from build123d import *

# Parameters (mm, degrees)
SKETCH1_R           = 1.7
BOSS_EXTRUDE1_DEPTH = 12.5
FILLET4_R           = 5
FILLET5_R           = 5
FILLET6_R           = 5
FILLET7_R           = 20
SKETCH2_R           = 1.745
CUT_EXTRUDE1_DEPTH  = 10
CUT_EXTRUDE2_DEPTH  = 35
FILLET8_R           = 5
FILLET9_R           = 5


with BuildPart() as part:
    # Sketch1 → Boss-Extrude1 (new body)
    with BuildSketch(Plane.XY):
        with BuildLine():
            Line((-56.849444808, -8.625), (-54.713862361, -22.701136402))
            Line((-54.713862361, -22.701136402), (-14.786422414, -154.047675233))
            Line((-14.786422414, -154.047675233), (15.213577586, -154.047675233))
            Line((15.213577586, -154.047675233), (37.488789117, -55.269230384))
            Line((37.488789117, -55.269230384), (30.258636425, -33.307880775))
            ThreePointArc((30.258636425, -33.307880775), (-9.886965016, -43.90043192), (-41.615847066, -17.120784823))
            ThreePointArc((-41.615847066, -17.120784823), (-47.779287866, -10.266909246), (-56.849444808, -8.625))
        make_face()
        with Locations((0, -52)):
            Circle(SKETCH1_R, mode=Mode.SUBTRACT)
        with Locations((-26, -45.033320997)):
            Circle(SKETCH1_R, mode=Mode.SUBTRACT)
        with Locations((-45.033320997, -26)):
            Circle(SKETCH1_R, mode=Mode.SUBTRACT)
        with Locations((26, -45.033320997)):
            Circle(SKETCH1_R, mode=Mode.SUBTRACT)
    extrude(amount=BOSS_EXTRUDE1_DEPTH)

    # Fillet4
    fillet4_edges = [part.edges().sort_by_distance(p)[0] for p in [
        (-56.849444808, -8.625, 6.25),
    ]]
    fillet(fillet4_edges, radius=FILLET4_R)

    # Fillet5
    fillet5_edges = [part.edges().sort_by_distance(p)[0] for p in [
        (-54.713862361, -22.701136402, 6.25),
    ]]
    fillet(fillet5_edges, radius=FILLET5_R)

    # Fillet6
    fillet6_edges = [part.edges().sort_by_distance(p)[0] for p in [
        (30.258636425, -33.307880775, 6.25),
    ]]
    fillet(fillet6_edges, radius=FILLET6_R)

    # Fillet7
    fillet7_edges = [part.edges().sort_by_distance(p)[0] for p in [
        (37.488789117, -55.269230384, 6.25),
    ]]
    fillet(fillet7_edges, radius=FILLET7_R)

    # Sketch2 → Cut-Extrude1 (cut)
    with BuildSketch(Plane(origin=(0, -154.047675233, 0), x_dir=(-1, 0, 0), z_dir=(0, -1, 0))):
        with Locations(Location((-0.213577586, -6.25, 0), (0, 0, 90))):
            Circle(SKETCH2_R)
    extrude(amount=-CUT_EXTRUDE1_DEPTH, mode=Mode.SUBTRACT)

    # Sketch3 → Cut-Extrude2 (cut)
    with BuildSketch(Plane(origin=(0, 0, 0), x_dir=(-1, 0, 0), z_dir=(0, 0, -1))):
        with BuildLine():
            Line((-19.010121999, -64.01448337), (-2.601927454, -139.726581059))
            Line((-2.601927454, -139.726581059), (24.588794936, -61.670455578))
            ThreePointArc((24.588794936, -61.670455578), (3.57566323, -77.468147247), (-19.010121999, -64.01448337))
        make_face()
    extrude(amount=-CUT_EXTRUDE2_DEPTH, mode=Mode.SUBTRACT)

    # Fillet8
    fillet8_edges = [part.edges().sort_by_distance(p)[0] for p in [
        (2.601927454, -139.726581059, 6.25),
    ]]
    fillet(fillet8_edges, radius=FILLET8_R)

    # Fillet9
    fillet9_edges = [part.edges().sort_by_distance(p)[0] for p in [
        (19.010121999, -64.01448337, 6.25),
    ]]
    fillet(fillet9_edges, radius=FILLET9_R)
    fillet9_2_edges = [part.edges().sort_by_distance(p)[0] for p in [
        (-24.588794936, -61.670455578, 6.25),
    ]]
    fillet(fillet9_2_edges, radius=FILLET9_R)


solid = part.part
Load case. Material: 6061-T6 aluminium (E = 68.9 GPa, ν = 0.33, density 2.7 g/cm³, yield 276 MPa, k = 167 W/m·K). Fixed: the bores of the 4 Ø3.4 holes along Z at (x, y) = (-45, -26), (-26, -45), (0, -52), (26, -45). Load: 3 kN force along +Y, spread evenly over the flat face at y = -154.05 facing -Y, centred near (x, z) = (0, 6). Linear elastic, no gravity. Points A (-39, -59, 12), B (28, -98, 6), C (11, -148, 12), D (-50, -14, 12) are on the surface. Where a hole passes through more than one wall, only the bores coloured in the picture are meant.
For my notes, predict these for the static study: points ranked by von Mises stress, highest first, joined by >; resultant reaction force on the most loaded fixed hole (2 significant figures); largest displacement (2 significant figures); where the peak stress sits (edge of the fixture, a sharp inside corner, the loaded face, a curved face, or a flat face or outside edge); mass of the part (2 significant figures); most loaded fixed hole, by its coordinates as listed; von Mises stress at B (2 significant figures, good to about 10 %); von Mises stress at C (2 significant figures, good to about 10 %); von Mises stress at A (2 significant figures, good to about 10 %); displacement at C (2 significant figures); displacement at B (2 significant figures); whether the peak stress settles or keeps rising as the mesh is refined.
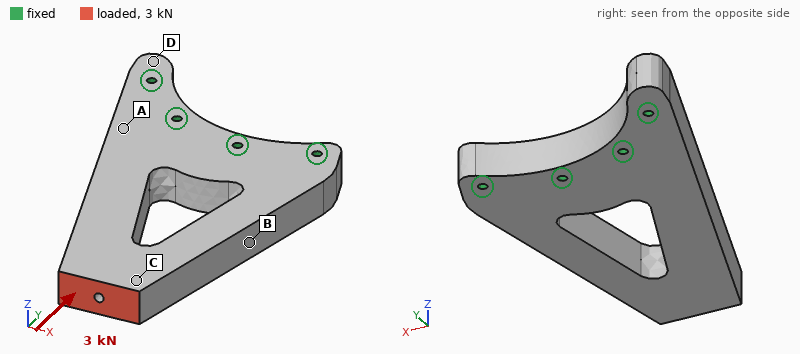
C > B > A > D
1.3 kN
13 µm
edge of the fixture
210 g
(26, -45)
6.0 MPa
7.8 MPa
3.3 MPa
12 µm
6.8 µm
keeps rising
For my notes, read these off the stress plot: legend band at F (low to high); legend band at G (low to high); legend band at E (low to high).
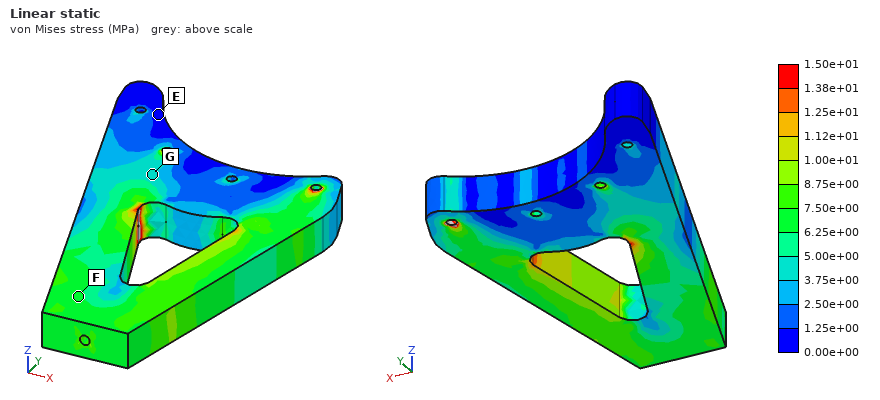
6.25e+00 to 7.50e+00 MPa
3.75e+00 to 5.00e+00 MPa
0.00e+00 to 1.25e+00 MPa
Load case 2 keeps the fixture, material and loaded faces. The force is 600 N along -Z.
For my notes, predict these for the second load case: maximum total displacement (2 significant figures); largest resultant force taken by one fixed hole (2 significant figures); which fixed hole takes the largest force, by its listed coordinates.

0.49 mm
1.1 kN
(0, -52)
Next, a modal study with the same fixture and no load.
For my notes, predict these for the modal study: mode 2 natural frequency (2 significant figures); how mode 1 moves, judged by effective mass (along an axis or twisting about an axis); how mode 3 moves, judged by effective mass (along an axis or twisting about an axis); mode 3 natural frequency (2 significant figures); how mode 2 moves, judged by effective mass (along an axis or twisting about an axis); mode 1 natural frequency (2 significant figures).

3800 Hz
along Z
along X
4000 Hz
twisting about Y
1000 Hz
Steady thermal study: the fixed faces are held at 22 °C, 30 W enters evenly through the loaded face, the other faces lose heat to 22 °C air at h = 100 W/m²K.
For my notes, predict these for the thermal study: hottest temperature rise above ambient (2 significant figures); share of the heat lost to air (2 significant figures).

28 K
47 %
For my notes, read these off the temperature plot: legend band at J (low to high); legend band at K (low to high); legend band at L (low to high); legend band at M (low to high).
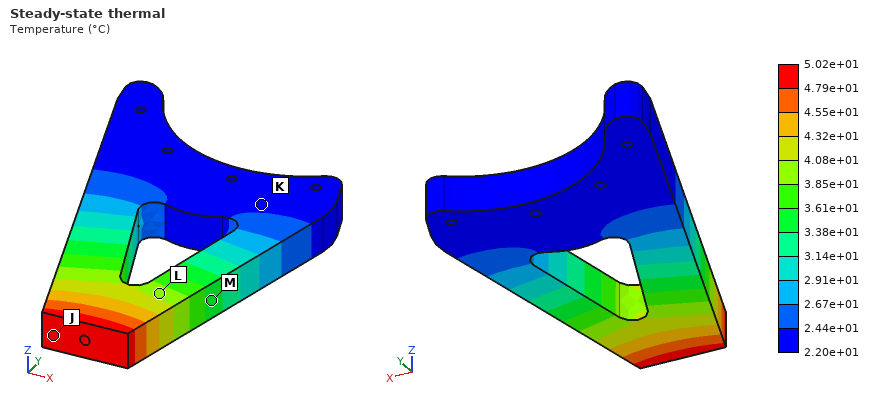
4.79e+01 to 5.02e+01 °C
2.20e+01 to 2.44e+01 °C
3.85e+01 to 4.08e+01 °C
3.38e+01 to 3.61e+01 °C
